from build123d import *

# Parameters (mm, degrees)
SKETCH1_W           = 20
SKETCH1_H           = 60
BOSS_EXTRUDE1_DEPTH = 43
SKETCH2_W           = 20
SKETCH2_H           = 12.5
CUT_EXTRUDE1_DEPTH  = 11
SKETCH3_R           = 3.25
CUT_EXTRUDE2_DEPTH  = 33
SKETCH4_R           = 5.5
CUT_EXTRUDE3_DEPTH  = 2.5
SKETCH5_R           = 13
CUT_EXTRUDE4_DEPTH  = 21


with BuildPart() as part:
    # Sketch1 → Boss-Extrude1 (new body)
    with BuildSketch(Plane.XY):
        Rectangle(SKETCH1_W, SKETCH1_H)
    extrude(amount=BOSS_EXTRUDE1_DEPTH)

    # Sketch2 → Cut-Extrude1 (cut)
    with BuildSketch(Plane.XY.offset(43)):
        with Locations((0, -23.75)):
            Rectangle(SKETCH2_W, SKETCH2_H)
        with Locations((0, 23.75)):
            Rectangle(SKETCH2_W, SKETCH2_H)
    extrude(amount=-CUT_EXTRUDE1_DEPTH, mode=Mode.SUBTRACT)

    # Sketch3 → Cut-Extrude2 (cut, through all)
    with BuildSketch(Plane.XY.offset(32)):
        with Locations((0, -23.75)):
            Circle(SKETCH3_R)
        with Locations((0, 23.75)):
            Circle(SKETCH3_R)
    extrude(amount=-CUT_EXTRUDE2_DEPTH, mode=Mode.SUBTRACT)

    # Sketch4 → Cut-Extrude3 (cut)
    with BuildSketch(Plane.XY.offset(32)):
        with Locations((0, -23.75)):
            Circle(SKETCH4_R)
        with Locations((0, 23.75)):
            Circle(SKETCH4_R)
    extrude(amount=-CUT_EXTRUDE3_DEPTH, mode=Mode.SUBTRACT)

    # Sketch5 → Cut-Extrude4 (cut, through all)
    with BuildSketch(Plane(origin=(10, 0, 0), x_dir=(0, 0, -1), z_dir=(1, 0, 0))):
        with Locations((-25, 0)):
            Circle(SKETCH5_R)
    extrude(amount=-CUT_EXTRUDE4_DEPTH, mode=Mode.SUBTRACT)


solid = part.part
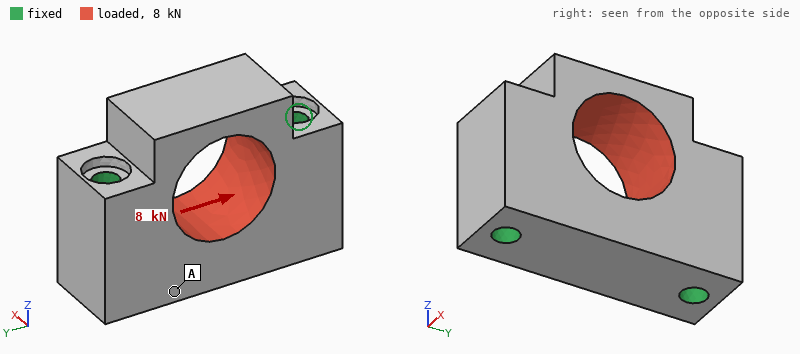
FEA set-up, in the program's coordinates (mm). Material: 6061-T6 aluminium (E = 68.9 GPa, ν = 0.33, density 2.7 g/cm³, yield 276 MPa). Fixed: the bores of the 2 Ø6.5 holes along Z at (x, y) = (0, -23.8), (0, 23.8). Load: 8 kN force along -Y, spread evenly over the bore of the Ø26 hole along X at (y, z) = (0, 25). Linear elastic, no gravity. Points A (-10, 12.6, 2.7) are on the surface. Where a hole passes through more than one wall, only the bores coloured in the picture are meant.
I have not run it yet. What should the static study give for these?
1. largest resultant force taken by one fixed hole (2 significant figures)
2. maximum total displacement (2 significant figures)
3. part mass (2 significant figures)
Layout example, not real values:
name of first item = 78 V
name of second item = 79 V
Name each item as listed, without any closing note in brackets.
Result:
largest resultant force taken by one fixed hole = 4.1 kN
maximum total displacement = 11 µm
part mass = 89 g
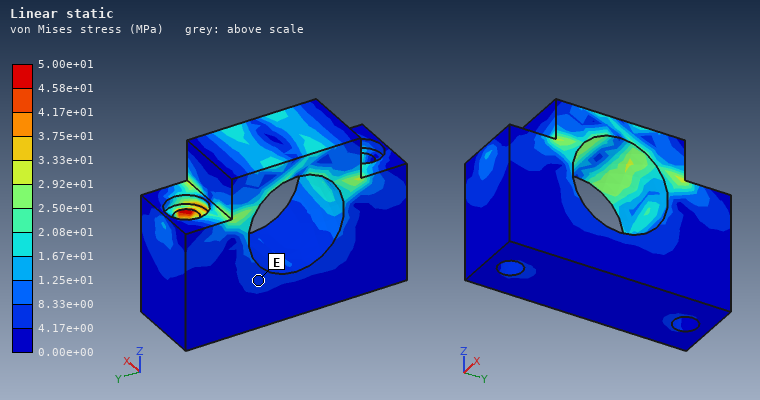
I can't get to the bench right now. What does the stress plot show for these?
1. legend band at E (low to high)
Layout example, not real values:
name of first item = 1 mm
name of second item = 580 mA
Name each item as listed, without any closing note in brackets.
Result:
legend band at E = 4.17e+00 to 8.33e+00 MPa
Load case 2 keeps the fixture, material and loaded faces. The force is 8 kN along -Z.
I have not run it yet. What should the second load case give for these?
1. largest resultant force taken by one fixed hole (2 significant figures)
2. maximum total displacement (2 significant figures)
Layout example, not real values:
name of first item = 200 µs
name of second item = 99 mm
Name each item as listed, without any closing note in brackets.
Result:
largest resultant force taken by one fixed hole = 4.1 kN
maximum total displacement = 9.8 µm
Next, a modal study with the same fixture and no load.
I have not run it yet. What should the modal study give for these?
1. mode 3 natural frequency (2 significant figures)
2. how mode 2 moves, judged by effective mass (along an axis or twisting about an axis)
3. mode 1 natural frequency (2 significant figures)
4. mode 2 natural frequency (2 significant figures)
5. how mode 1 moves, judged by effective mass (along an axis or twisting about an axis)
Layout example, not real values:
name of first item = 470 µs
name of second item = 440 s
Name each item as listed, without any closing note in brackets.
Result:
mode 3 natural frequency = 24 kHz
how mode 2 moves, judged by effective mass = along Y
mode 1 natural frequency = 15 kHz
mode 2 natural frequency = 21 kHz
how mode 1 moves, judged by effective mass = along X
